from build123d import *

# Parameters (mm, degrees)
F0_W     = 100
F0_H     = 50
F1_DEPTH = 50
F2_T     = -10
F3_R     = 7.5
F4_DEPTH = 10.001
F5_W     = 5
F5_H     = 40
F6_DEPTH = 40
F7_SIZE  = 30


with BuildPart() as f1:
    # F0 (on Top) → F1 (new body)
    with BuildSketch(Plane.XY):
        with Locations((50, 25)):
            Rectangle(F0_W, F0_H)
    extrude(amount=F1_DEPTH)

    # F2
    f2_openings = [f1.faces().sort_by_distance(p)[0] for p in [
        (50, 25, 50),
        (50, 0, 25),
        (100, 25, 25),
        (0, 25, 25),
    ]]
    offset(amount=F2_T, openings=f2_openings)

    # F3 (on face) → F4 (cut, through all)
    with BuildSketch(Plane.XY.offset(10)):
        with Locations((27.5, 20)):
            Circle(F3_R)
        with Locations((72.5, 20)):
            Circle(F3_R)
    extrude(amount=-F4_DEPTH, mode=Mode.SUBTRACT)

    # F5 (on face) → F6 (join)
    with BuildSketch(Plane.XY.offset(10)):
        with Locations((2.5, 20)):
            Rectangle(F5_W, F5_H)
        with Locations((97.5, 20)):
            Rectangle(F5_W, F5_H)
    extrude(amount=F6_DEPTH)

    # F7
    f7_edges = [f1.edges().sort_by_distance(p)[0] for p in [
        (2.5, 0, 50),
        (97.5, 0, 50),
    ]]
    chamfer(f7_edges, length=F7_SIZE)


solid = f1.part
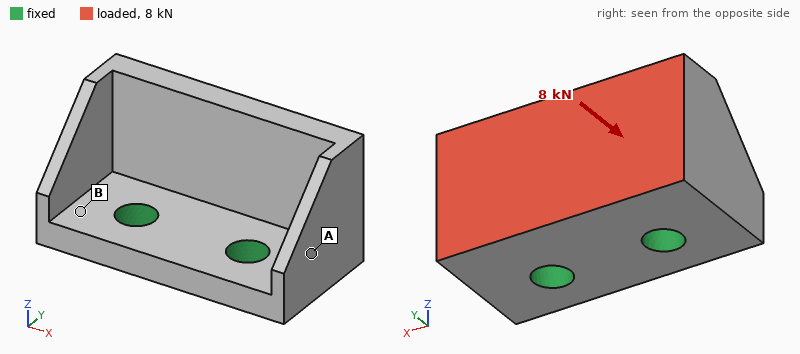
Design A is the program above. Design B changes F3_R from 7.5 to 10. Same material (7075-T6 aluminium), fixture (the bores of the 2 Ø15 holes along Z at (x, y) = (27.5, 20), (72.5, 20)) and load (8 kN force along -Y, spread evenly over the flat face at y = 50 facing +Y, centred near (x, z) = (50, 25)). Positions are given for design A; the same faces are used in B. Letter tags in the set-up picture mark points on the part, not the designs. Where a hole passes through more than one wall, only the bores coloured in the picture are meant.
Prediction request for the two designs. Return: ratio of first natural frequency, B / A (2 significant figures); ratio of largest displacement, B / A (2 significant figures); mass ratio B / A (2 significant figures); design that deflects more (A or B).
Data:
1.1
0.84
0.97
A
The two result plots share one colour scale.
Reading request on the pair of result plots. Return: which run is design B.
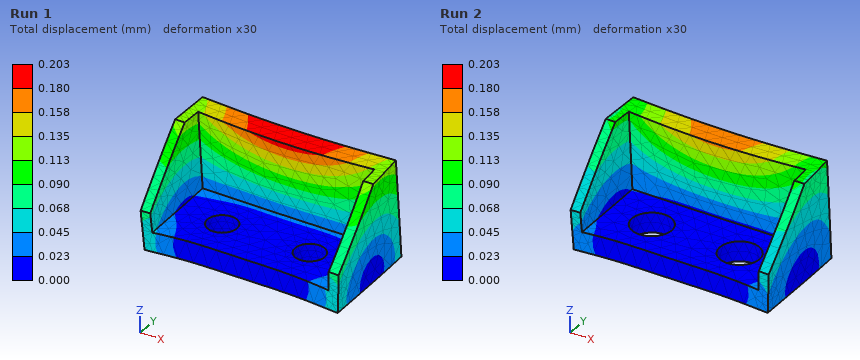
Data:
Run 2
